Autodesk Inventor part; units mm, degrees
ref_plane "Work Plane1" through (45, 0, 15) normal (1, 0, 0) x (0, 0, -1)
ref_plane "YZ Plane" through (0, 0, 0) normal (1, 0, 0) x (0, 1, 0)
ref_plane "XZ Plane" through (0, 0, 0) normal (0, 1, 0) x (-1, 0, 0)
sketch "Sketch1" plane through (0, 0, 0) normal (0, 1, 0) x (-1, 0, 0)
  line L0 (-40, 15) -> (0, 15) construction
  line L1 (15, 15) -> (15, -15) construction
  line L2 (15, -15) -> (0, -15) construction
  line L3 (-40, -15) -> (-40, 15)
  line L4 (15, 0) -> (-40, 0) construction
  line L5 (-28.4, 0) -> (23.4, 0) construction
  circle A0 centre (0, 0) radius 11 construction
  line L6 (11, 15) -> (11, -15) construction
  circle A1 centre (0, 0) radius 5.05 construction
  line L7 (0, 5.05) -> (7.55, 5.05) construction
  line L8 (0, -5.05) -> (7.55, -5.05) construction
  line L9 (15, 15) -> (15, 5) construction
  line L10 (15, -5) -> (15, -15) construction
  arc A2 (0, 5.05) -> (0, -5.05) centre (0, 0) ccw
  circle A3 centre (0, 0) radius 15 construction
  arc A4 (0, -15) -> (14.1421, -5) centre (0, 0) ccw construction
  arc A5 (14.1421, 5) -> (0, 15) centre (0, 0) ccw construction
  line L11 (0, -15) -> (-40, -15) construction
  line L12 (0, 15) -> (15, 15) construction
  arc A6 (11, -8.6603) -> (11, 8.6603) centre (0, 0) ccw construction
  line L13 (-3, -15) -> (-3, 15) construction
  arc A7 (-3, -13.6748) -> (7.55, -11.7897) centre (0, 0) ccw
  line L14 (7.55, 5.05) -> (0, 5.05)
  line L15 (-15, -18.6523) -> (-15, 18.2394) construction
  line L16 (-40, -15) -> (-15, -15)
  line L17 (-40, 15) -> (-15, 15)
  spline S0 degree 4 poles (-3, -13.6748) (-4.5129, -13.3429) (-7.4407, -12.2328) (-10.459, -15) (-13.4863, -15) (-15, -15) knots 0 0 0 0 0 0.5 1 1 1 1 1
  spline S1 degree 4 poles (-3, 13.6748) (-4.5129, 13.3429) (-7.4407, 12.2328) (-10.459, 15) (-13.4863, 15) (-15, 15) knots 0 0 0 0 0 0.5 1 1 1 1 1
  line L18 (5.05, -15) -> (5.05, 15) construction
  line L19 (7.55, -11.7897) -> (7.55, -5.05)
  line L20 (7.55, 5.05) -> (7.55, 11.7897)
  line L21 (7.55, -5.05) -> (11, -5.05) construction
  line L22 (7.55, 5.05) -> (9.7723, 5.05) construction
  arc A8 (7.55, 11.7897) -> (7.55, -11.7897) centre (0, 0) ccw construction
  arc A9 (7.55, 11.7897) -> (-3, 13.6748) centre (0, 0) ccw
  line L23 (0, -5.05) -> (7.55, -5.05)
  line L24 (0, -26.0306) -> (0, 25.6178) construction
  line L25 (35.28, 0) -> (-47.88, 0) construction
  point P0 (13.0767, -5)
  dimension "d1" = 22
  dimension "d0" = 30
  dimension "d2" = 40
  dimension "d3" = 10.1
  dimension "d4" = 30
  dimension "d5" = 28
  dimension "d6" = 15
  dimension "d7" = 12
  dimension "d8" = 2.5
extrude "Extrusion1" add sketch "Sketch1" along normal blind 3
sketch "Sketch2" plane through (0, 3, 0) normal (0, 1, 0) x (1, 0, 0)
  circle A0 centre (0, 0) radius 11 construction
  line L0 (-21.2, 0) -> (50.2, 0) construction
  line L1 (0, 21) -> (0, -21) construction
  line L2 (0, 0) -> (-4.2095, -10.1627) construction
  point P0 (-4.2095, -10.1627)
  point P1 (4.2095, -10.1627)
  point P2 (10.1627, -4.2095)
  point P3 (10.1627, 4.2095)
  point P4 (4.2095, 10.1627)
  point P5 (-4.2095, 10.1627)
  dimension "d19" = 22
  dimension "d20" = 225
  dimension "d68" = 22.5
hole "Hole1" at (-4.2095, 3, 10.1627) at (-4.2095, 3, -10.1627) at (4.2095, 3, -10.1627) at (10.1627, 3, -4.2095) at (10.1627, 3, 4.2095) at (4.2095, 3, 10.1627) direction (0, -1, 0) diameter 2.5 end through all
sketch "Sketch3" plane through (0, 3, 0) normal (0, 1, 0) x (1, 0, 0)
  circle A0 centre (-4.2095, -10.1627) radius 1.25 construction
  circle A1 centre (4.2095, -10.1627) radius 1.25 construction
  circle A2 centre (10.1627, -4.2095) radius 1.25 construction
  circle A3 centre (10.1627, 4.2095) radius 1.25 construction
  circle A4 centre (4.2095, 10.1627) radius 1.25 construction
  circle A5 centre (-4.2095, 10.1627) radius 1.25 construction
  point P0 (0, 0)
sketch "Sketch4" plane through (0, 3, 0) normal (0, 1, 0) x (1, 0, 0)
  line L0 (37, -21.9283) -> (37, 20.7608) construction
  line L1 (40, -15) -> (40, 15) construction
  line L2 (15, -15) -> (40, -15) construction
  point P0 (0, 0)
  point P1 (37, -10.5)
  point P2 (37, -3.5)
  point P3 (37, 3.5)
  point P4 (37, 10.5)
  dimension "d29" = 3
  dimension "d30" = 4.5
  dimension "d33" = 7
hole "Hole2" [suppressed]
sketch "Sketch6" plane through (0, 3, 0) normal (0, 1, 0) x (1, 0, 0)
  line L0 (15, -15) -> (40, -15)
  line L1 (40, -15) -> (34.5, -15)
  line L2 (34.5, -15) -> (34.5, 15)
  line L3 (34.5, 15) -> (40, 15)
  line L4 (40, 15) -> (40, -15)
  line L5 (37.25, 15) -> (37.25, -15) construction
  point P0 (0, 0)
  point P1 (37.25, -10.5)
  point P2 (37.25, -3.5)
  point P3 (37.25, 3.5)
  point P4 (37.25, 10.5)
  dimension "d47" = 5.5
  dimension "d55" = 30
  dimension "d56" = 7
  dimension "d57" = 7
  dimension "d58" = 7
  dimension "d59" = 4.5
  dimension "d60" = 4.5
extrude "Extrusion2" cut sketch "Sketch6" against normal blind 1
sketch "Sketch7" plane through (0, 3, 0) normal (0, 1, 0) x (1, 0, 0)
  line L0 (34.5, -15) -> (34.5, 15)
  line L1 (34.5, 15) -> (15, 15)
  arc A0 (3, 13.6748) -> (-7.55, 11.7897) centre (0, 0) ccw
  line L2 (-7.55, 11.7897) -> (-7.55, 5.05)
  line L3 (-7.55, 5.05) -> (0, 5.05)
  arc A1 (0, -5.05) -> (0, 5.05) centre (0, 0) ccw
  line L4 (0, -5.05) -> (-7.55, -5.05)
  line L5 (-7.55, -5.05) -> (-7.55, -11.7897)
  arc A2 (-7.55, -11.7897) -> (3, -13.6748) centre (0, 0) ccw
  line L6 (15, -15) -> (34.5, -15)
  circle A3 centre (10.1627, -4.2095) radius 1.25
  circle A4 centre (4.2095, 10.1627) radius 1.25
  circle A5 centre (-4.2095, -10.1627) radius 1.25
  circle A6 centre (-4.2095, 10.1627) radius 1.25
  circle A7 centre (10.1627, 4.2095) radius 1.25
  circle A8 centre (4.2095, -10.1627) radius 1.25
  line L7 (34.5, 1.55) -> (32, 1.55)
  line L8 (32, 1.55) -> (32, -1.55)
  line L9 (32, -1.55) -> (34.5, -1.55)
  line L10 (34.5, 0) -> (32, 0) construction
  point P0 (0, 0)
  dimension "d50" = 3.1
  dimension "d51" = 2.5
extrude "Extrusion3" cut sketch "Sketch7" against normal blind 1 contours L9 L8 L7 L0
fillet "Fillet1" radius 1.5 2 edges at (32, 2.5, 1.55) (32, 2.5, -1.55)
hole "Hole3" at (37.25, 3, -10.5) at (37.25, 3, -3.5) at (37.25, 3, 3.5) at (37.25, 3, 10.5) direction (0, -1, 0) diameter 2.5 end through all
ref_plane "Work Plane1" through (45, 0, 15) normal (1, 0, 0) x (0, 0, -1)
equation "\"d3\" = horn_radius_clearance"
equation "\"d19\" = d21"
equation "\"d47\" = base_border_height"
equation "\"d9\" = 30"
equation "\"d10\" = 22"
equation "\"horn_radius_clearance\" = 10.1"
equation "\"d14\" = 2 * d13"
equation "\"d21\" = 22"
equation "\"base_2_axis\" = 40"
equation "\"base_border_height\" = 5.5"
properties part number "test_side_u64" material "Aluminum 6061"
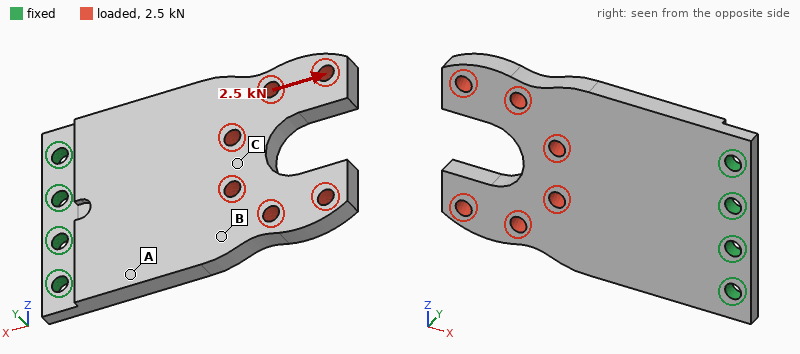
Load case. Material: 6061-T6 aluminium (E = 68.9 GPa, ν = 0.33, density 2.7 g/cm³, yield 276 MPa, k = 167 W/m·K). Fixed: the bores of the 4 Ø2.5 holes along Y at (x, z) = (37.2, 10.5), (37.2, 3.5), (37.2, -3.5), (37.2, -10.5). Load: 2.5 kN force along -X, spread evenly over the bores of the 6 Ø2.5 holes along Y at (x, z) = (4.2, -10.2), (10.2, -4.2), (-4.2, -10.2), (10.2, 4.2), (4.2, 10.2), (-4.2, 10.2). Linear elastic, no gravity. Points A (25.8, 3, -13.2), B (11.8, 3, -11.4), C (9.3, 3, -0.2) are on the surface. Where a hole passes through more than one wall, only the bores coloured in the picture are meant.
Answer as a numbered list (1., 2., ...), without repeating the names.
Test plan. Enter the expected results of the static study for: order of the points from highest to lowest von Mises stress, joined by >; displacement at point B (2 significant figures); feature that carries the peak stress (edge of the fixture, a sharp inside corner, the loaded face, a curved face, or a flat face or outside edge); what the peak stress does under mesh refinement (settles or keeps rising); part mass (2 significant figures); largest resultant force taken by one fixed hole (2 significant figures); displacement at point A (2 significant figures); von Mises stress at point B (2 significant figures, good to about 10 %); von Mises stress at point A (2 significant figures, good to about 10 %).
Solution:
1. B > A > C
2. 0.060 mm
3. edge of the fixture
4. keeps rising
5. 9.3 g
6. 690 N
7. 0.026 mm
8. 33 MPa
9. 26 MPa
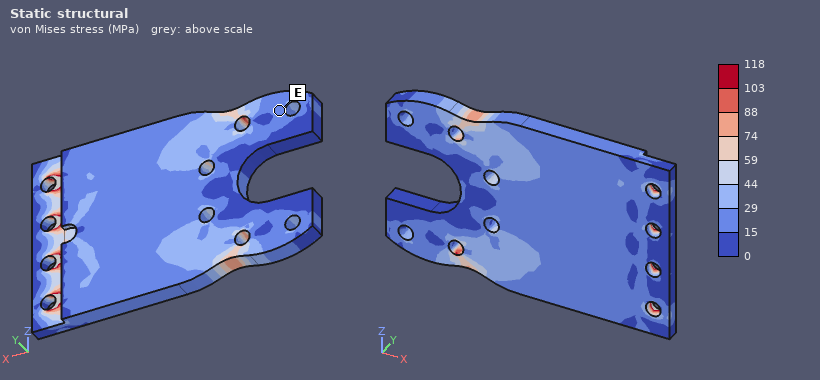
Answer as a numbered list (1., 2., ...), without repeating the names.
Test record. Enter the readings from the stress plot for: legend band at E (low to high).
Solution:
1. 15 to 29 MPa
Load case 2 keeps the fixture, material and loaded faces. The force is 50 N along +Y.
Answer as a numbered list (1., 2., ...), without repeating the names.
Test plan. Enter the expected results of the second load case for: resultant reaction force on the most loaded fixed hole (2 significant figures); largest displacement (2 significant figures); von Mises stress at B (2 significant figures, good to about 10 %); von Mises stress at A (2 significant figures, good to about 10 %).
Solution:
1. 25 N
2. 0.29 mm
3. 11 MPa
4. 26 MPa
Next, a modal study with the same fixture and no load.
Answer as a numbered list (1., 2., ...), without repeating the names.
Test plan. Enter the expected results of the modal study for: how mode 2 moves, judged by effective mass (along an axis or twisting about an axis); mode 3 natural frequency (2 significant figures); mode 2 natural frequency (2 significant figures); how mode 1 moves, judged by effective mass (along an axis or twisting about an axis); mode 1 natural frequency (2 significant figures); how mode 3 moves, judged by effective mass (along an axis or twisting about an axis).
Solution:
1. twisting about X
2. 7300 Hz
3. 3800 Hz
4. along Y
5. 1300 Hz
6. along Y
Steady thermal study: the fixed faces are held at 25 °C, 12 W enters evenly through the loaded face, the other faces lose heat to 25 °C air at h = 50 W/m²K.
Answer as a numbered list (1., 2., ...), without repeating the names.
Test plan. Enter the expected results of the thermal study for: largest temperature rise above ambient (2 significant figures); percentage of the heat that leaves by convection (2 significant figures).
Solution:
1. 29 K
2. 17 %
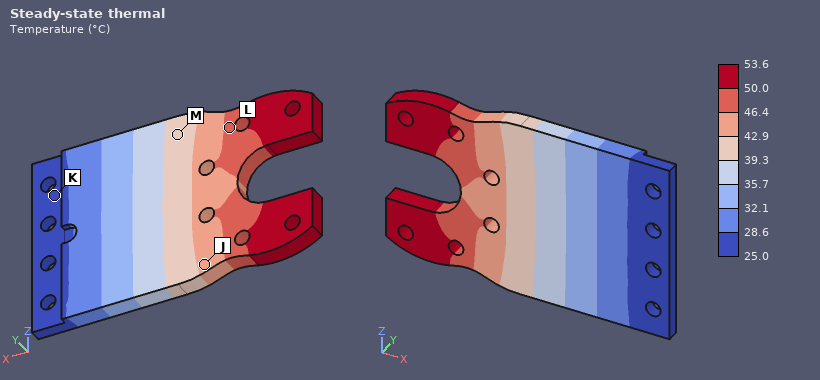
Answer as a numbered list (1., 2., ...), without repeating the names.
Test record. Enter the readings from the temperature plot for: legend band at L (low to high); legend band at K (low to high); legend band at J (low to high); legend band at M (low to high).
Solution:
1. 46.4 to 50.0 °C
2. 25.0 to 28.6 °C
3. 42.9 to 46.4 °C
4. 39.3 to 42.9 °C
